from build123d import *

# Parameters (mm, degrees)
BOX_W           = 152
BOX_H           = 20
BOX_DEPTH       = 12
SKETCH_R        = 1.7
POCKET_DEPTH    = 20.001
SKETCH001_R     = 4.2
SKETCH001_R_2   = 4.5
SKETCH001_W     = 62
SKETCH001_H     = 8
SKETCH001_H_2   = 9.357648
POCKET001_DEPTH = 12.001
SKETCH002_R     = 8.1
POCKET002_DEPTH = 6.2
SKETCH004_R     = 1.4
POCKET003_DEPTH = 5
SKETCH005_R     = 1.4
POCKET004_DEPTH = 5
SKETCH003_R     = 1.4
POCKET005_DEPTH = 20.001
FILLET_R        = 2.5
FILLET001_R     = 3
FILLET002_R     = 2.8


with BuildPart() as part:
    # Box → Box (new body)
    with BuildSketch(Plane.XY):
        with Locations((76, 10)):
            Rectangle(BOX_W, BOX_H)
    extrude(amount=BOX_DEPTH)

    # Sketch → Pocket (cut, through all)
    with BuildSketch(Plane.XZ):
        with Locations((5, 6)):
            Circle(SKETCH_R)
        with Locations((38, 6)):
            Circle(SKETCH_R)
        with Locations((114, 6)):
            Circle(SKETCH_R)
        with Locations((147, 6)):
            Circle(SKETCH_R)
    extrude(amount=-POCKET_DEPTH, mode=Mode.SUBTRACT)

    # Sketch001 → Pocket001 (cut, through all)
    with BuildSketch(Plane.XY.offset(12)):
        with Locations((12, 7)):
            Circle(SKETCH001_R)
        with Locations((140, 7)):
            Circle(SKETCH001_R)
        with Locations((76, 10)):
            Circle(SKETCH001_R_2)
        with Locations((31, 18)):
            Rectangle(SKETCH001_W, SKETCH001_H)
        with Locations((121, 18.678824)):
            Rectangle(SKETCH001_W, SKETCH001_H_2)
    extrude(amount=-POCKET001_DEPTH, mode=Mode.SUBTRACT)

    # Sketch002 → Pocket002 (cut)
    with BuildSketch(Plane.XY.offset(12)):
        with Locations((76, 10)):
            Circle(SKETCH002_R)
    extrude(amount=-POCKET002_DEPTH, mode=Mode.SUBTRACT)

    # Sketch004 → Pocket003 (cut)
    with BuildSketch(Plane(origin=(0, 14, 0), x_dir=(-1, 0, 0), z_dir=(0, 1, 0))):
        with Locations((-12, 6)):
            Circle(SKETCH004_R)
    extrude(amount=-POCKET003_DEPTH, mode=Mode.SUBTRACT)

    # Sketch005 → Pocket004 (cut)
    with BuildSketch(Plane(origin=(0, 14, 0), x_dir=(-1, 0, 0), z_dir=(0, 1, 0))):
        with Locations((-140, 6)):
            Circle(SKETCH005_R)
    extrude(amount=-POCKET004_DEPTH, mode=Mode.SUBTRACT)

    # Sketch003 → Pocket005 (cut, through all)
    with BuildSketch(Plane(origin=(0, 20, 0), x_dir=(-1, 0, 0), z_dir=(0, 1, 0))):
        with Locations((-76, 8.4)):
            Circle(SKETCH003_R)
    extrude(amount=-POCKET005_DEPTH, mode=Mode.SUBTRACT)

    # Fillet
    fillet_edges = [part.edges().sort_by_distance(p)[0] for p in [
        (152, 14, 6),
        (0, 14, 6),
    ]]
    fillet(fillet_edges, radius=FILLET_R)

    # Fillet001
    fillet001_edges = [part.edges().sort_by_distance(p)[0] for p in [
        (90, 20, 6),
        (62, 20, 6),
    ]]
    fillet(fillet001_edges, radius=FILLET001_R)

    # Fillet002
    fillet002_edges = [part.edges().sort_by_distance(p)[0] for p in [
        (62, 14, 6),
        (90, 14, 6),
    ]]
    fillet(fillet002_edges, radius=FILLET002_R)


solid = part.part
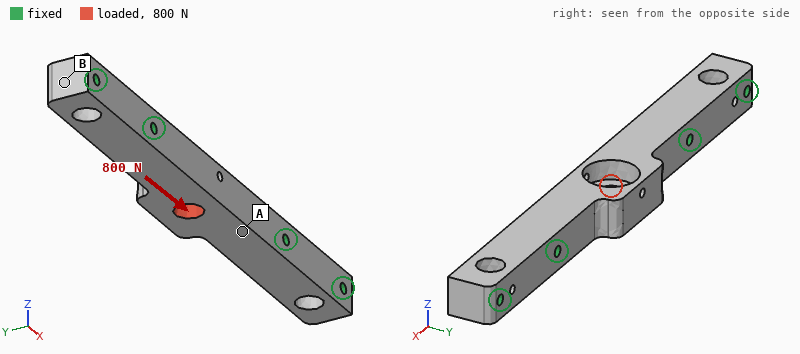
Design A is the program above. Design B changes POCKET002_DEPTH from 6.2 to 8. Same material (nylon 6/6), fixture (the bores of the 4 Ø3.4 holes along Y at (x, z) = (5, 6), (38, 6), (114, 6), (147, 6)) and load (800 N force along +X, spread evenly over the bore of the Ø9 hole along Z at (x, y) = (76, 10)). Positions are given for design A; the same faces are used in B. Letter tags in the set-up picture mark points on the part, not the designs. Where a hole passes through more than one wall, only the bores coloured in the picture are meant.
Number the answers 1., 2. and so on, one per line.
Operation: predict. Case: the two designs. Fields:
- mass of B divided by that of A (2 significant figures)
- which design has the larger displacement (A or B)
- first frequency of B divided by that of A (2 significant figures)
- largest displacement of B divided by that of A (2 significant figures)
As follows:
1. 0.99
2. B
3. 1.0
4. 1.2
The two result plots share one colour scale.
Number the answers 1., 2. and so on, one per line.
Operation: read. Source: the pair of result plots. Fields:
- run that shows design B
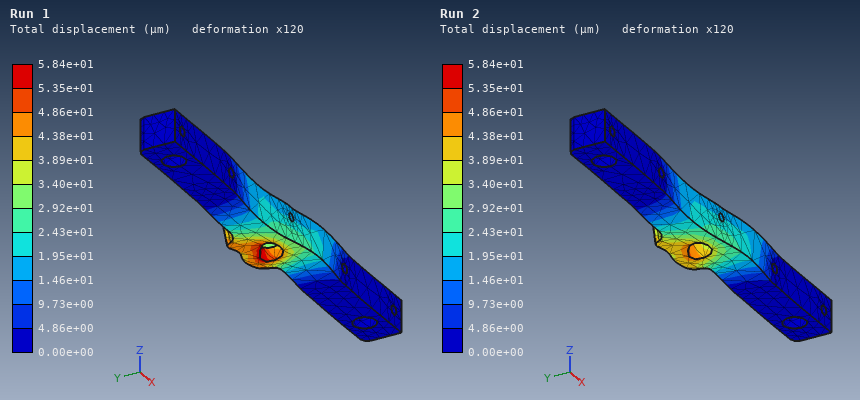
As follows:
1. Run 1
